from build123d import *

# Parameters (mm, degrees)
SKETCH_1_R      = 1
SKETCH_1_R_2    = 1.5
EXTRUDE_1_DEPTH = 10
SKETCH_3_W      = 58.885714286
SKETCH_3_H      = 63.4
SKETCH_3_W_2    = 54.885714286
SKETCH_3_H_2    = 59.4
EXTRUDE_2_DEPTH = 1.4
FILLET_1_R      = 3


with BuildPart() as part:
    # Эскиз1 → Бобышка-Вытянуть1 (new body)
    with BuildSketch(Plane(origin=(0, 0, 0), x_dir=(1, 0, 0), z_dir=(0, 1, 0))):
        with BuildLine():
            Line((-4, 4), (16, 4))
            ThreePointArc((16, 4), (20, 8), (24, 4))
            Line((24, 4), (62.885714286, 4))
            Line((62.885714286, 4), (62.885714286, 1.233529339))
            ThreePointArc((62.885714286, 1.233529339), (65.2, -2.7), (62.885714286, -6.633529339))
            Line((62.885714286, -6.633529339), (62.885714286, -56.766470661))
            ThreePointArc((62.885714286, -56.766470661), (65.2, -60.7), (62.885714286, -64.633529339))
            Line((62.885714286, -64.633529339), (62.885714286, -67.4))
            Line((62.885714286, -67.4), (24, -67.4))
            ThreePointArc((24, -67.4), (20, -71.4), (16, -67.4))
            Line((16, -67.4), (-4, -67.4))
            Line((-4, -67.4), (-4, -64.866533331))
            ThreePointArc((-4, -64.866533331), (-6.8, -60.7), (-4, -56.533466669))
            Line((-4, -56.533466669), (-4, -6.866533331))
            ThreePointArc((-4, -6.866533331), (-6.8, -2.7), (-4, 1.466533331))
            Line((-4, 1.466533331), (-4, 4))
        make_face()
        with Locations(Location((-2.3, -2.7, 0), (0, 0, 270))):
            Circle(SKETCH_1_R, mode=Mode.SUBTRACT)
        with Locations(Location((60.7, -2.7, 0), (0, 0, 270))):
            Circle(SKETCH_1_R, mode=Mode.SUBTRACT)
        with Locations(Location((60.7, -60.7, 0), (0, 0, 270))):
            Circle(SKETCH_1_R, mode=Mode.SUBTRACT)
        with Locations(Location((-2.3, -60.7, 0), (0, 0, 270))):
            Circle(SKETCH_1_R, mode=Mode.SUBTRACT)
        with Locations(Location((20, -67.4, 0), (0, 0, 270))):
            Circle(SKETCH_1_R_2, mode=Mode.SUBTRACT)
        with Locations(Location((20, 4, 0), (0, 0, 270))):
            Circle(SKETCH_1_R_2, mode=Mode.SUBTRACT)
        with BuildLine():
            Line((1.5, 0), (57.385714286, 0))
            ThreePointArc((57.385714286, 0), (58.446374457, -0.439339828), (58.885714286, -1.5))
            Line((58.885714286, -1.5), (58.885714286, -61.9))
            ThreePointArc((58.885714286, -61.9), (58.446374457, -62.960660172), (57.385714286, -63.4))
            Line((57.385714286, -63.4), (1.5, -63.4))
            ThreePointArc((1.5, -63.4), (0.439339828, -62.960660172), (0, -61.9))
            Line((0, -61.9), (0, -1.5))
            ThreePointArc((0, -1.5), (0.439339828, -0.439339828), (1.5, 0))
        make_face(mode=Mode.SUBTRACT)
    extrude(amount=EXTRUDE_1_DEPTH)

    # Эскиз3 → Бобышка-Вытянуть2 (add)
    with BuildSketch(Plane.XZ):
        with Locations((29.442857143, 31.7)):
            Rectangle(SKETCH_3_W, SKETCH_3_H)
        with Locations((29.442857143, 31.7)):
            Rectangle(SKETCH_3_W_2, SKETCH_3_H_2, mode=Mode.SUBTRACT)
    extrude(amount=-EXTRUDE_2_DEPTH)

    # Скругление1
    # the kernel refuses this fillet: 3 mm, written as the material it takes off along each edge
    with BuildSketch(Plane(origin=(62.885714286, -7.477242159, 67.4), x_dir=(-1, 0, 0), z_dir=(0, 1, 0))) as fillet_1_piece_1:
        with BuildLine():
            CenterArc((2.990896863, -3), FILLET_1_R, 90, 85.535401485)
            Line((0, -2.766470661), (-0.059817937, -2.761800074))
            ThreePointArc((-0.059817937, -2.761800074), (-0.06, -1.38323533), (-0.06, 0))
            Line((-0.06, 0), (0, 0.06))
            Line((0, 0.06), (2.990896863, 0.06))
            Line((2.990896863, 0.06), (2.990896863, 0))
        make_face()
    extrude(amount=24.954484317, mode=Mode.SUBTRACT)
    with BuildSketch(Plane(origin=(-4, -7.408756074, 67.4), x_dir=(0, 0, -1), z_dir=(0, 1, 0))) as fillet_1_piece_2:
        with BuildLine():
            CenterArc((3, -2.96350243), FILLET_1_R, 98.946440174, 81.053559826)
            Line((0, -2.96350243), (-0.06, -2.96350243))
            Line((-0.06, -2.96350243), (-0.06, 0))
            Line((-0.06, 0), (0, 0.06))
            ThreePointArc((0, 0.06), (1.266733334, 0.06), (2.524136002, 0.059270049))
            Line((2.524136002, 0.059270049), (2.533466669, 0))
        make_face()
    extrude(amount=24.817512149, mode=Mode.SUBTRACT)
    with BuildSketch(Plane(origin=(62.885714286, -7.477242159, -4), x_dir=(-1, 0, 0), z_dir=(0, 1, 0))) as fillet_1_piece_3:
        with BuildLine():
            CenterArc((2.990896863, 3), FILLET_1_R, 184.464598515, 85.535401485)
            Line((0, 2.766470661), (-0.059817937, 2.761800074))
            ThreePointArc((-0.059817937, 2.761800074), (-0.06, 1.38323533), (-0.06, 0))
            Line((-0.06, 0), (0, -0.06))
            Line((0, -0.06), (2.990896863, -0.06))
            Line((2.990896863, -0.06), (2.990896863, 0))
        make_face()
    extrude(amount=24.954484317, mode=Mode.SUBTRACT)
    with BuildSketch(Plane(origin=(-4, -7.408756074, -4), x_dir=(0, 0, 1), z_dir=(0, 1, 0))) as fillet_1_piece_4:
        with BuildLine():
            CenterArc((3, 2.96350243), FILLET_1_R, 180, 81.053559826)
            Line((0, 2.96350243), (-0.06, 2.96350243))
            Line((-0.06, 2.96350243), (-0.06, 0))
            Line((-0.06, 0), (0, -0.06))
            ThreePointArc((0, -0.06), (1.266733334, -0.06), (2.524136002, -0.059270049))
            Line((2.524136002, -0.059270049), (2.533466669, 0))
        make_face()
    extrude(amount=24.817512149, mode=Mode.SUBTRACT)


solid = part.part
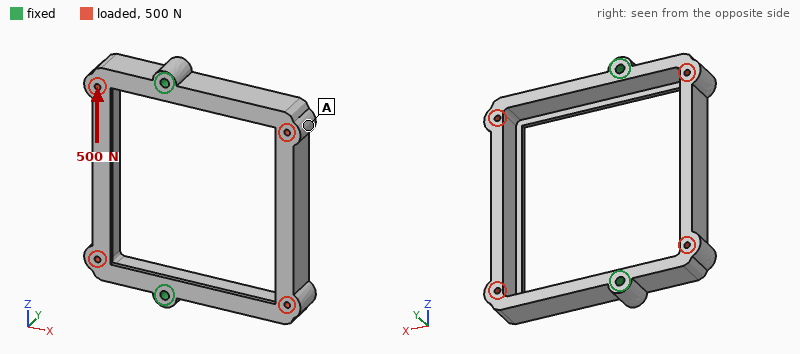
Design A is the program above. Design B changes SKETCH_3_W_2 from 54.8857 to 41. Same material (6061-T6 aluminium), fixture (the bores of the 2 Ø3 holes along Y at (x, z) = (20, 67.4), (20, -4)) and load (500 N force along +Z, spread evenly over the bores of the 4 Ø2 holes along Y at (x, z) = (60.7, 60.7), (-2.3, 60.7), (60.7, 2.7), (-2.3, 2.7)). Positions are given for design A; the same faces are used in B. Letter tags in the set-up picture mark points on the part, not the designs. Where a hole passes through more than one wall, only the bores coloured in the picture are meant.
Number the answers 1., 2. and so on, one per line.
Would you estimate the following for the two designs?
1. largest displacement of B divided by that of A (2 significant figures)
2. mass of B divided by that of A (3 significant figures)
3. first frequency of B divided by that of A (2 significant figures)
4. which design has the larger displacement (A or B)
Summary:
1. 0.54
2. 1.10
3. 1.2
4. A
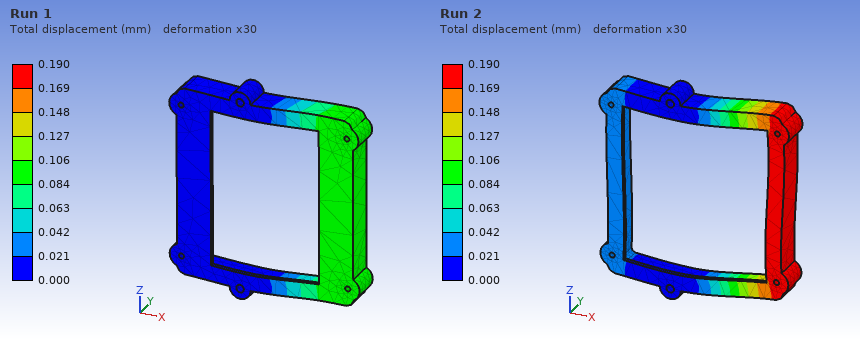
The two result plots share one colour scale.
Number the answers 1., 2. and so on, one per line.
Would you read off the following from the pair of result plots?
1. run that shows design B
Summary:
1. Run 1
